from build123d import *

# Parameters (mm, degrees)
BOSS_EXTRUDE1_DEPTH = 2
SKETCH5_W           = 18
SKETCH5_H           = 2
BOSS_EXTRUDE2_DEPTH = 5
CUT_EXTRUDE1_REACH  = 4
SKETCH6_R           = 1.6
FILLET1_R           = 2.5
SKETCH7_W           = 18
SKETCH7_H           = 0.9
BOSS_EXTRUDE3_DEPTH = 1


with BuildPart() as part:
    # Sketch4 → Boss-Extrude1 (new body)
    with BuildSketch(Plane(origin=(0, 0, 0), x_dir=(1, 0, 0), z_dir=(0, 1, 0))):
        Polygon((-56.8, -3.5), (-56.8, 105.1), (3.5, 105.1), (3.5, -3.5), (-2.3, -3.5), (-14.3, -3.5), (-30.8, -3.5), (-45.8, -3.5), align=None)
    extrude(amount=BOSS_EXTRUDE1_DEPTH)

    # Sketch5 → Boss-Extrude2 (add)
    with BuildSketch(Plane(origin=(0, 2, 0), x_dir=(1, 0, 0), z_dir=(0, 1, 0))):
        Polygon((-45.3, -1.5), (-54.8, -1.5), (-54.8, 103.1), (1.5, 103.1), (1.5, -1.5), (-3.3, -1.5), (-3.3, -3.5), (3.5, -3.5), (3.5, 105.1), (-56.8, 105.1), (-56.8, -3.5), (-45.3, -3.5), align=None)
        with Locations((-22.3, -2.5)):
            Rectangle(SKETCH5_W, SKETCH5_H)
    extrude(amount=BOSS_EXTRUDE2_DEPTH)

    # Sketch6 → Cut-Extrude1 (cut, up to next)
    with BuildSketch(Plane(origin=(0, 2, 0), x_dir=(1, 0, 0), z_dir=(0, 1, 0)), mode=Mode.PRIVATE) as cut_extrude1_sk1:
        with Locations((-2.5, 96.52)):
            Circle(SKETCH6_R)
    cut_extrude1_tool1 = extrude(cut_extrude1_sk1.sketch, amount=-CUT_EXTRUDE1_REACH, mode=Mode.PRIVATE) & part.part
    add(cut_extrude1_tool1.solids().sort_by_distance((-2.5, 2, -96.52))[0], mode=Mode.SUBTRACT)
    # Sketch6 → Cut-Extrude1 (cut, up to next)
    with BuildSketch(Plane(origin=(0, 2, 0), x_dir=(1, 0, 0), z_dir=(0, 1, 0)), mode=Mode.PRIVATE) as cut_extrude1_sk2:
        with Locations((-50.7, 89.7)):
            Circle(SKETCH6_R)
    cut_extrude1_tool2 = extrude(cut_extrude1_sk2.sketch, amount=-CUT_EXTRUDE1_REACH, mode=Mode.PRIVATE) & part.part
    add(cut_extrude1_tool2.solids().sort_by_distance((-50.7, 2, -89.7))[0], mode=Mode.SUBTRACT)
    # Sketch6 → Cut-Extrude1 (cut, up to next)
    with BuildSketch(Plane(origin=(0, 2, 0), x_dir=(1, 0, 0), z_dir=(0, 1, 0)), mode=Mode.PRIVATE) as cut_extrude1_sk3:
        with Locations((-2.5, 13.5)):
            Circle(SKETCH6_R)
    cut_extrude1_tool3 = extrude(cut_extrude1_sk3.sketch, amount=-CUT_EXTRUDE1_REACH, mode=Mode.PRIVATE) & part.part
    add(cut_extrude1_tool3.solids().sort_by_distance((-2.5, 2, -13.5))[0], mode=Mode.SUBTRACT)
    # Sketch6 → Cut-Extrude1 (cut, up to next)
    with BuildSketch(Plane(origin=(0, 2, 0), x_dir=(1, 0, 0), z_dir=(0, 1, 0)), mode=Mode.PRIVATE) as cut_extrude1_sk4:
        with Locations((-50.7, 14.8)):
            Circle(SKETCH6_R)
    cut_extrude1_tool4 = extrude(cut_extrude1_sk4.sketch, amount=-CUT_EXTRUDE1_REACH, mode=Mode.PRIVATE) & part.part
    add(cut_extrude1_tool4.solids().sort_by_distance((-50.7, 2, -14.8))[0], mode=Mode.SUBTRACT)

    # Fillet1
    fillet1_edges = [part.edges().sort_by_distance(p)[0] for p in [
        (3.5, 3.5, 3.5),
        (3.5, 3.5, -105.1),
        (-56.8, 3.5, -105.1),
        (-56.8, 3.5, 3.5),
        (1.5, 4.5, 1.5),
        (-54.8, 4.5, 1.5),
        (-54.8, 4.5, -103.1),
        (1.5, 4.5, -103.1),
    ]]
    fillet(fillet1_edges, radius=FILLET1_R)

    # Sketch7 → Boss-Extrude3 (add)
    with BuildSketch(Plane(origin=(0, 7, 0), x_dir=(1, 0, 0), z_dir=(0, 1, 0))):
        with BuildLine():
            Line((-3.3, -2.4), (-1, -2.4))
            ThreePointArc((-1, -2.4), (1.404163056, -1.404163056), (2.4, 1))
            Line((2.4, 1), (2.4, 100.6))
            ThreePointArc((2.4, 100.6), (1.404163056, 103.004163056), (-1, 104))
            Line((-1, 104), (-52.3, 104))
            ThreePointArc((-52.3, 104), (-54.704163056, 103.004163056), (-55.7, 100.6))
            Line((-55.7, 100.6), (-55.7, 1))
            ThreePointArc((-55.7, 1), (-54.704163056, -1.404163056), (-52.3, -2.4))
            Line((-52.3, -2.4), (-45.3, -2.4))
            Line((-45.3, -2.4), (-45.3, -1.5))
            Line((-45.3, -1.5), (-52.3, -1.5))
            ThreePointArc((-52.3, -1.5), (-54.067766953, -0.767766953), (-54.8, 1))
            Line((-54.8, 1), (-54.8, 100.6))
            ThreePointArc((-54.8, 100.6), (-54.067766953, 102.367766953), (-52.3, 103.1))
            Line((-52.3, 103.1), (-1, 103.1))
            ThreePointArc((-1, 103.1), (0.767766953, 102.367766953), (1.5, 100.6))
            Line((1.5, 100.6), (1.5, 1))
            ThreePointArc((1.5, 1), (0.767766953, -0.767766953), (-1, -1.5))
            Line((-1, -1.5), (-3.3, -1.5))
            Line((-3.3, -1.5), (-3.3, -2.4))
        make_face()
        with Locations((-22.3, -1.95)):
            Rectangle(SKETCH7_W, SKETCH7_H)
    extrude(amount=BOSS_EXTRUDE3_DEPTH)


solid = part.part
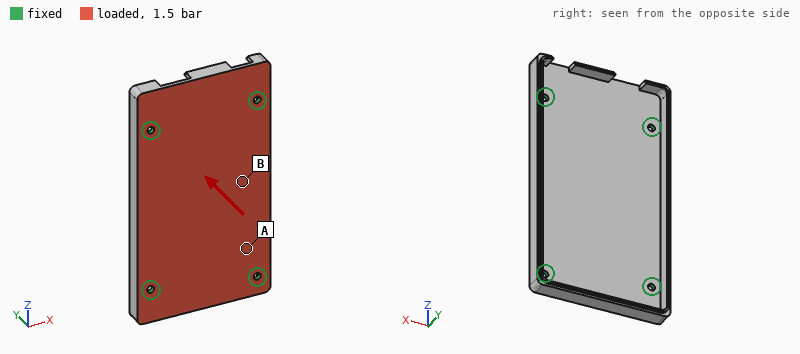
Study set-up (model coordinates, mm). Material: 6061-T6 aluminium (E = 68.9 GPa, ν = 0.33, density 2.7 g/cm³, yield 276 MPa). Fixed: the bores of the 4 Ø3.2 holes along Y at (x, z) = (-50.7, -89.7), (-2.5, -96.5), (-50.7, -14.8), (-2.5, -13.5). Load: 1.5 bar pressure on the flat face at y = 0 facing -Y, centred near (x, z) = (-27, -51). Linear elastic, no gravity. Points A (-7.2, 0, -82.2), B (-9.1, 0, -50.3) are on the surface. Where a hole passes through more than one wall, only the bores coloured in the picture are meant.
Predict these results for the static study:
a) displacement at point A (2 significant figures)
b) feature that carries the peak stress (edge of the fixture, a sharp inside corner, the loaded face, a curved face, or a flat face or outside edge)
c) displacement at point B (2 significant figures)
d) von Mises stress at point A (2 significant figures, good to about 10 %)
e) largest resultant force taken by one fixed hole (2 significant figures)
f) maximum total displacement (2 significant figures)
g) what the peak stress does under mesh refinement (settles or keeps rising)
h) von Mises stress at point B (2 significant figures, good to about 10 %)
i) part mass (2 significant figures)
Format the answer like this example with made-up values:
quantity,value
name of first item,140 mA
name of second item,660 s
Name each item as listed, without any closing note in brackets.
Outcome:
quantity,value
displacement at point A,0.076 mm
feature that carries the peak stress,edge of the fixture
displacement at point B,0.17 mm
von Mises stress at point A,14 MPa
largest resultant force taken by one fixed hole,290 N
maximum total displacement,0.23 mm
what the peak stress does under mesh refinement,keeps rising
von Mises stress at point B,30 MPa
part mass,44 g
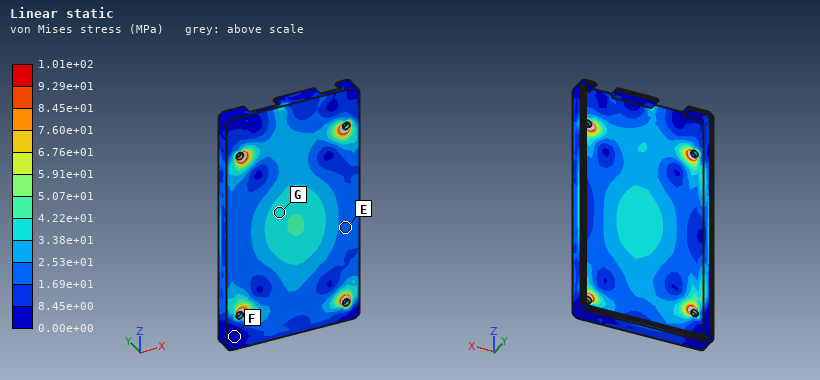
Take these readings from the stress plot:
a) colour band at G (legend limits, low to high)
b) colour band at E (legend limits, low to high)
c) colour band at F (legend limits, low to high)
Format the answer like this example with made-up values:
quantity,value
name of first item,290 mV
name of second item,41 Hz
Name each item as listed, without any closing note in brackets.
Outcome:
quantity,value
colour band at G,3.38e+01 to 4.22e+01 MPa
colour band at E,1.69e+01 to 2.53e+01 MPa
colour band at F,0.00e+00 to 8.45e+00 MPa
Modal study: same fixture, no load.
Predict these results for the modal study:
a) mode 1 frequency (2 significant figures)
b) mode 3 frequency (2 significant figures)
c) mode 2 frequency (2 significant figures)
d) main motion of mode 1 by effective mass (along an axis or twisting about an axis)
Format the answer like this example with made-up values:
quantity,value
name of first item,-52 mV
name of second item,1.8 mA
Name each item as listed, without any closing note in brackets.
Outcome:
quantity,value
mode 1 frequency,2100 Hz
mode 3 frequency,3600 Hz
mode 2 frequency,3500 Hz
main motion of mode 1 by effective mass,along Y
